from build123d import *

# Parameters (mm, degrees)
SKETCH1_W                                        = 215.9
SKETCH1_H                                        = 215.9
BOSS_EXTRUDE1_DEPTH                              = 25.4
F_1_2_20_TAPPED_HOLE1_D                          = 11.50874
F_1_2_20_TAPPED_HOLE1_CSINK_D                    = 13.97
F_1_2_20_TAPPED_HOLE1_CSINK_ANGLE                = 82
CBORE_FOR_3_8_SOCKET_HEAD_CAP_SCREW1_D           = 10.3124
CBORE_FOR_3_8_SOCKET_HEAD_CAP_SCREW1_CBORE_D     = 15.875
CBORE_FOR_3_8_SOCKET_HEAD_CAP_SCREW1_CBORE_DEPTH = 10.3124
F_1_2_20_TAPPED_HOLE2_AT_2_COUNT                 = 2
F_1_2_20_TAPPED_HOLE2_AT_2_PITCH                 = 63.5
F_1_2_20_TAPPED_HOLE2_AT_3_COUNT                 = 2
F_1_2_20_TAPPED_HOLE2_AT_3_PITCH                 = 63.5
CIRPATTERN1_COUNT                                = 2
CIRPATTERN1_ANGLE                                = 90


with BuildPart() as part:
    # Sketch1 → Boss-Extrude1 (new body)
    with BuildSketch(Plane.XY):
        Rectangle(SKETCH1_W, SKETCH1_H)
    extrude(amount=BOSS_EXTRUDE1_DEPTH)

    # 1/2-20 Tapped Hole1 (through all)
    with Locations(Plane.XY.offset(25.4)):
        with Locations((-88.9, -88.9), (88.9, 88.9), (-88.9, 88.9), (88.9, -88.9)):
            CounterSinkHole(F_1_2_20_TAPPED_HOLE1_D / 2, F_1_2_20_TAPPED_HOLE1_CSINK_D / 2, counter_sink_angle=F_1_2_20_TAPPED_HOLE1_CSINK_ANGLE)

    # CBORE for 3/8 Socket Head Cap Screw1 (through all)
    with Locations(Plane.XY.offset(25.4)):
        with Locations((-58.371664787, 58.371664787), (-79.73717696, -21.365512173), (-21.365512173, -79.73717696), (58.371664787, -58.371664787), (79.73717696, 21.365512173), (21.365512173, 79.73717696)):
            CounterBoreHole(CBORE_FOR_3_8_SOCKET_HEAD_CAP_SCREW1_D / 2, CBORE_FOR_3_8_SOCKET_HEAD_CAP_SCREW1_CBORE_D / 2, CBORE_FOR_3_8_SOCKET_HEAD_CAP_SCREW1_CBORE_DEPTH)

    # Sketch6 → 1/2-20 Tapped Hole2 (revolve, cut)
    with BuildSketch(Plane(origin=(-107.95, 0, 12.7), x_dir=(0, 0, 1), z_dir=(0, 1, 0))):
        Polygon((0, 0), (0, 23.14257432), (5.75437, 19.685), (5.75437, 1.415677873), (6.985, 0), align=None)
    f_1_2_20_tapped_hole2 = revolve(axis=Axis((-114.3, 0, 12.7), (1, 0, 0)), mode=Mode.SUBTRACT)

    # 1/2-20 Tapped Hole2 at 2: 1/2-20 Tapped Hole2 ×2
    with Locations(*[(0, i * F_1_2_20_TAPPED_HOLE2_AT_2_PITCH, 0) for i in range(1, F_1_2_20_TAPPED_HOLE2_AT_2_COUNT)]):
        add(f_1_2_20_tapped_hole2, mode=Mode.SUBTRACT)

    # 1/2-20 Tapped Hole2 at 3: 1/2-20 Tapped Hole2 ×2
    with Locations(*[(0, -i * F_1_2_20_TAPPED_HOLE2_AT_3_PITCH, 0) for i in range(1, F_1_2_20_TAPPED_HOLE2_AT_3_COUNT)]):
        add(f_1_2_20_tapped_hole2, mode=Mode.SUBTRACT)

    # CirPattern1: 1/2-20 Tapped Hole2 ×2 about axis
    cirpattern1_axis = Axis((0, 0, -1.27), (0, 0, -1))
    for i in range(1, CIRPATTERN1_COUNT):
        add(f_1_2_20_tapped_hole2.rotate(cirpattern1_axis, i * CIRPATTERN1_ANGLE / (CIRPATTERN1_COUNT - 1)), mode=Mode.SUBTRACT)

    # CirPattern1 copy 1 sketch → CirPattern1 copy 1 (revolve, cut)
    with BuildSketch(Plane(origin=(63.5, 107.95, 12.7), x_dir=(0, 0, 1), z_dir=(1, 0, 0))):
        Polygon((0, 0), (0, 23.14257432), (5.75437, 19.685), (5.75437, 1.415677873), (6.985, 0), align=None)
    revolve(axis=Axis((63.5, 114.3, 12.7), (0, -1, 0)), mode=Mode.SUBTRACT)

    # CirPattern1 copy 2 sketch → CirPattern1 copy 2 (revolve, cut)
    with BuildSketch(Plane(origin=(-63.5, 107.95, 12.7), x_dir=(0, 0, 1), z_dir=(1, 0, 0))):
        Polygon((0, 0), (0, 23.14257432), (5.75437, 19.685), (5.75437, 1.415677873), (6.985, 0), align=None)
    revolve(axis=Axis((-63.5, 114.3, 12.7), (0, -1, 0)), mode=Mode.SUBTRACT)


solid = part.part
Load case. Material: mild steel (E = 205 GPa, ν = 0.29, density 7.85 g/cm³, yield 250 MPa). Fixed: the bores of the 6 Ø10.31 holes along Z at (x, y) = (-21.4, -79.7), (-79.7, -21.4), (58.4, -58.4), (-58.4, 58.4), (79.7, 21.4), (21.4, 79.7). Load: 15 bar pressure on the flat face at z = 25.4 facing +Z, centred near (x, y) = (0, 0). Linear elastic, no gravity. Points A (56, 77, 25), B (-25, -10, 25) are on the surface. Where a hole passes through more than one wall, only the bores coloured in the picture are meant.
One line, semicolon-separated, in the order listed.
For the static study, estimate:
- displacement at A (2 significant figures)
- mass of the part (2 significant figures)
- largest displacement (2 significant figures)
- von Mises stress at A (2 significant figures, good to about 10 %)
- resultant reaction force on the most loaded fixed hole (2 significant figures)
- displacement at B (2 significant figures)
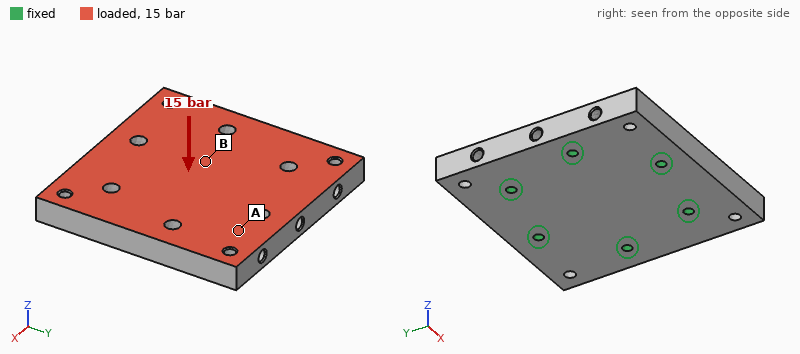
6.4 µm; 9.0 kg; 20 µm; 12 MPa; 12 kN; 5.1 µm
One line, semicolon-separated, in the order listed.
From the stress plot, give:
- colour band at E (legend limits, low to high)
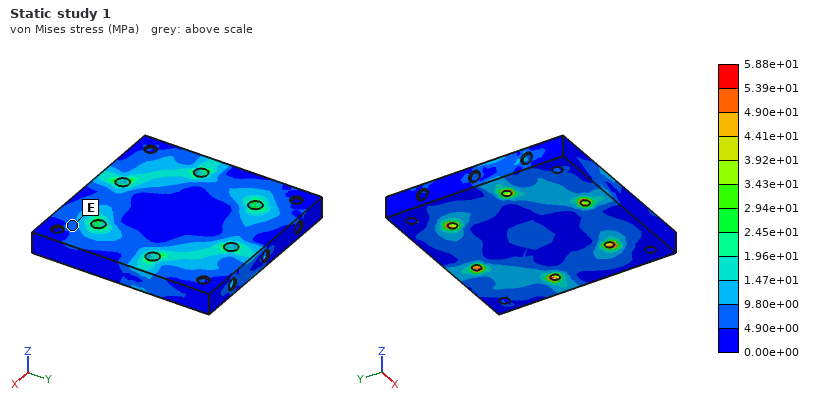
4.90e+00 to 9.80e+00 MPa
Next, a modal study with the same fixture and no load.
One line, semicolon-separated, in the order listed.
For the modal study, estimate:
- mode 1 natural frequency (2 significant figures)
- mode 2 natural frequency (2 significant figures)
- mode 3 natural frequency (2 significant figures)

3800 Hz; 3900 Hz; 4500 Hz
